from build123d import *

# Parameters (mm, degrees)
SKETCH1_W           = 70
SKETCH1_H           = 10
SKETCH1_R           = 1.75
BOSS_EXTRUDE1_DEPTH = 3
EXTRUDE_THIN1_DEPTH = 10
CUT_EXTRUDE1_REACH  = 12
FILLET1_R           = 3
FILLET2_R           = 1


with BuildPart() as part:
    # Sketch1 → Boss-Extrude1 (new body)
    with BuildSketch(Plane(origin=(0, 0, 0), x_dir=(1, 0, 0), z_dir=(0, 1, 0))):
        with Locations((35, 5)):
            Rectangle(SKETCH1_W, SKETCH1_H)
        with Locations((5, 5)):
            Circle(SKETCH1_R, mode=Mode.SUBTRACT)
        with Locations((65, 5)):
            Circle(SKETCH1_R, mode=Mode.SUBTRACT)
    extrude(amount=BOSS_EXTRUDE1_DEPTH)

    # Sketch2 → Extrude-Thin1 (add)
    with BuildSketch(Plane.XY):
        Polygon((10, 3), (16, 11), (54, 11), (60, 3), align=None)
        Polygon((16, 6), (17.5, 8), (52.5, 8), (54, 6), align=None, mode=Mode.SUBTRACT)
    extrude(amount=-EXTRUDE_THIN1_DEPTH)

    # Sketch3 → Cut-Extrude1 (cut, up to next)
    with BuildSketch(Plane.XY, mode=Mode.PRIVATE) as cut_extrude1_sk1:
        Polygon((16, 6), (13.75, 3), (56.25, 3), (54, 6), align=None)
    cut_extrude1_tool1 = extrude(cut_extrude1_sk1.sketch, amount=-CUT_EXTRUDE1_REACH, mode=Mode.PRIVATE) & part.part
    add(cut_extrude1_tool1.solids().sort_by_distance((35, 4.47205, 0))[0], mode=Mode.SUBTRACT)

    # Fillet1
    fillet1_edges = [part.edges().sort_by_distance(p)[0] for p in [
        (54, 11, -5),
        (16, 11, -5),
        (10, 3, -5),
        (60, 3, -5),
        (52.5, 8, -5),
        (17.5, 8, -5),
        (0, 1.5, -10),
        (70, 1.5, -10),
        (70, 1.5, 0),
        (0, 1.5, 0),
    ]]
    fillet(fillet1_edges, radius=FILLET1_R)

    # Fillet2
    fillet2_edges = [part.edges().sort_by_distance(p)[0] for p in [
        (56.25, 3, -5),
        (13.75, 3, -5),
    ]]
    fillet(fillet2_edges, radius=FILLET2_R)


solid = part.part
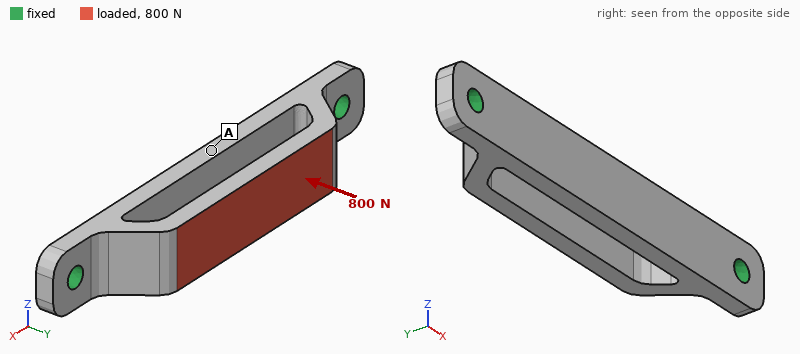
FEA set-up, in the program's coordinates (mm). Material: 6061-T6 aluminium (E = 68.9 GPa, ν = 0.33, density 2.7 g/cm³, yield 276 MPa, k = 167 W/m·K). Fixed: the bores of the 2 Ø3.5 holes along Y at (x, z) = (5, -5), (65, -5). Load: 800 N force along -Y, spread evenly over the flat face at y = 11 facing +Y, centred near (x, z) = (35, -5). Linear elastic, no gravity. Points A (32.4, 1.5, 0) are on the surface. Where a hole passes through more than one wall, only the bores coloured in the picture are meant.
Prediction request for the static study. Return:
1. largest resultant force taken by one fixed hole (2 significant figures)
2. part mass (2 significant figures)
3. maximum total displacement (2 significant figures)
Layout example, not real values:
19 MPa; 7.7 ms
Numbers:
680 N; 9.8 g; 0.12 mm
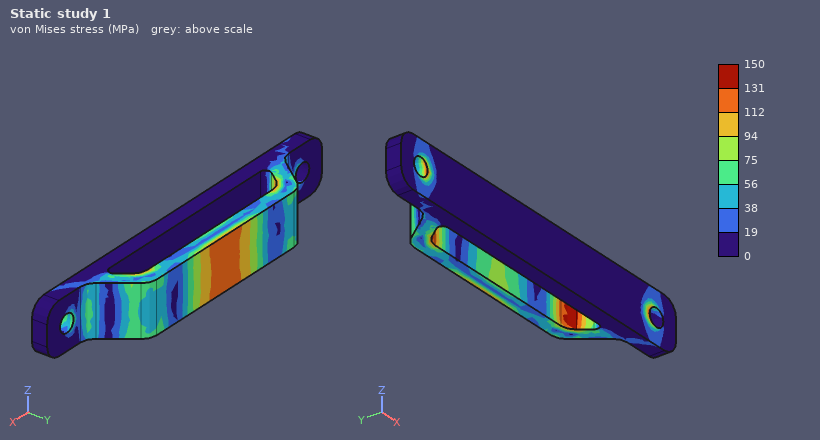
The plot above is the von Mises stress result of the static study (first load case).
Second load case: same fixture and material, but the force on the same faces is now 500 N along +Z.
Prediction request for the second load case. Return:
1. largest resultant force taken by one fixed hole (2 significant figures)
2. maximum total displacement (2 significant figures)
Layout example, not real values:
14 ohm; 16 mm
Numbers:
250 N; 87 µm
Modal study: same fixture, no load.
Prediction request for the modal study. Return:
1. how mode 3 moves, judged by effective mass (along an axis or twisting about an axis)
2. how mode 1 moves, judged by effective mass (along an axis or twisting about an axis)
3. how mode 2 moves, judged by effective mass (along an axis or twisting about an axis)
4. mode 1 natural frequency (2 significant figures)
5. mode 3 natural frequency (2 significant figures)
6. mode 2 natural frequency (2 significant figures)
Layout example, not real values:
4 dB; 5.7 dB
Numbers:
along Y; along Y; along Z; 6700 Hz; 8800 Hz; 7200 Hz
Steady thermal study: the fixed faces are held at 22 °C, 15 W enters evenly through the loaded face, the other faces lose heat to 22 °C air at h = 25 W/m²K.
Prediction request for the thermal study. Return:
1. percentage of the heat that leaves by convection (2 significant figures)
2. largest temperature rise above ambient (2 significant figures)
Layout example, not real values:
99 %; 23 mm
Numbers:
5.6 %; 33 K
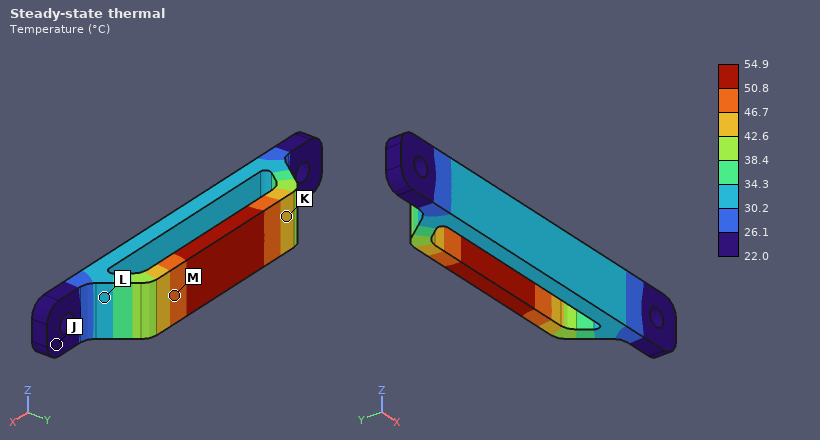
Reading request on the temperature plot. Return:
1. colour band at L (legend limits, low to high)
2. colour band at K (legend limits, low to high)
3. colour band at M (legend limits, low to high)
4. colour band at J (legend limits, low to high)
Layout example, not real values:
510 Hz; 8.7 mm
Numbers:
30.2 to 34.3 °C; 42.6 to 46.7 °C; 46.7 to 50.8 °C; 22.0 to 26.1 °C
